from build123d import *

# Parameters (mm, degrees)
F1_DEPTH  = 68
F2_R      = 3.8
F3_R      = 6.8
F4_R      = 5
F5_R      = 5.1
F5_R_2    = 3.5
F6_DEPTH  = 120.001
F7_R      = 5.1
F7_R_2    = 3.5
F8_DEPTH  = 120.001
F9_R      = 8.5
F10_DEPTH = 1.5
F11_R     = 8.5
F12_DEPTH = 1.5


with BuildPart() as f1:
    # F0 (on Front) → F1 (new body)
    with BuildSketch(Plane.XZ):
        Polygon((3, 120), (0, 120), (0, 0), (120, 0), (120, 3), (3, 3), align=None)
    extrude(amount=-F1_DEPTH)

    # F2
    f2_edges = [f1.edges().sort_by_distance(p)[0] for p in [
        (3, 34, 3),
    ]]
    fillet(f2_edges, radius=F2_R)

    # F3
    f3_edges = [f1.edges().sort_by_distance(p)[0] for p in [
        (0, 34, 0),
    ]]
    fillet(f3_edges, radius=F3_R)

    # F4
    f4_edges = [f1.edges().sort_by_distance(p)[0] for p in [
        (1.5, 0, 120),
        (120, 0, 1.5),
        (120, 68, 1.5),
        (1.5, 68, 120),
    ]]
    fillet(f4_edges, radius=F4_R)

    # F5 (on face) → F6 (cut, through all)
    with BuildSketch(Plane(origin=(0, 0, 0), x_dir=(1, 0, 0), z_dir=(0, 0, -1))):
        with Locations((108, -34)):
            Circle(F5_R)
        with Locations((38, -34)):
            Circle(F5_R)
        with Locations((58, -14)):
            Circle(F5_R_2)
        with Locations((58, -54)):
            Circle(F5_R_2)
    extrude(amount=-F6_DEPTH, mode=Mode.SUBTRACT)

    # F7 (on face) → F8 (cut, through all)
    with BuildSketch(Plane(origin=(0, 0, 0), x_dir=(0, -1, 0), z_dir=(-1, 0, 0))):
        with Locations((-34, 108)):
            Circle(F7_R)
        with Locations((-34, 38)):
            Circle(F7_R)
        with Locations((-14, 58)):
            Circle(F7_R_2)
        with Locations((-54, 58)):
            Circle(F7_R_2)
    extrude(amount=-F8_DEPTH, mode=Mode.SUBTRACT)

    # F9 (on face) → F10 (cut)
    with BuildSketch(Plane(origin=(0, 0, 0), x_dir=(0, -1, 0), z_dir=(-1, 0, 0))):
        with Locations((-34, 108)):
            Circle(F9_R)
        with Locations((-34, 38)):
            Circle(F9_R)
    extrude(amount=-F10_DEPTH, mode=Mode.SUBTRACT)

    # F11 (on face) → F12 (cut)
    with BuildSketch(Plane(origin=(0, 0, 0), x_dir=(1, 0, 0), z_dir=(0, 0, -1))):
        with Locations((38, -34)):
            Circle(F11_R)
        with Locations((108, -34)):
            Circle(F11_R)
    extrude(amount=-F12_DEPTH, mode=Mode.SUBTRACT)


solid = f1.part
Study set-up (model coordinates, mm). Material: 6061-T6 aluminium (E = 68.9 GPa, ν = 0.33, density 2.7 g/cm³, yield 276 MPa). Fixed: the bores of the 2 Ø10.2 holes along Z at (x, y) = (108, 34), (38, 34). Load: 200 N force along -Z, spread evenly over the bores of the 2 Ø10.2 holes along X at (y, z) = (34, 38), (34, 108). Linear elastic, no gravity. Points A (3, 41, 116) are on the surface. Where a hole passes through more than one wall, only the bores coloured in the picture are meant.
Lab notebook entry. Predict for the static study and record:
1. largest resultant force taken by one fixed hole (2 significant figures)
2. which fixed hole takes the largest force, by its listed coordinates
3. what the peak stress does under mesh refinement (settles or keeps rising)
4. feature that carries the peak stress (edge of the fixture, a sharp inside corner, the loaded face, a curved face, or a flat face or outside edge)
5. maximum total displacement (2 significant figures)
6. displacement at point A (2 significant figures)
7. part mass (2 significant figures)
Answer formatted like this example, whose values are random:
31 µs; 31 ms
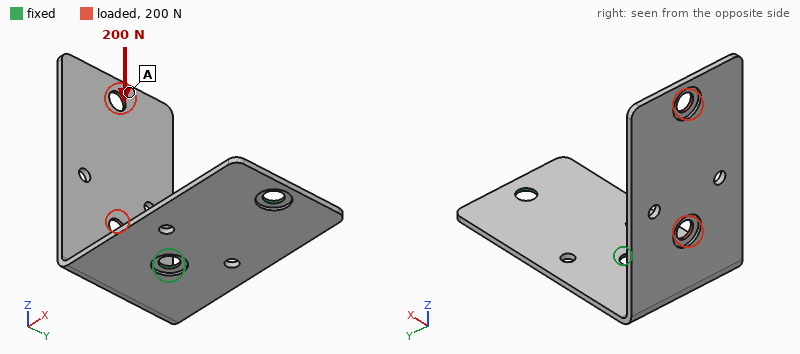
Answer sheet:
490 N; (38, 34); keeps rising; edge of the fixture; 1.9 mm; 1.8 mm; 120 g
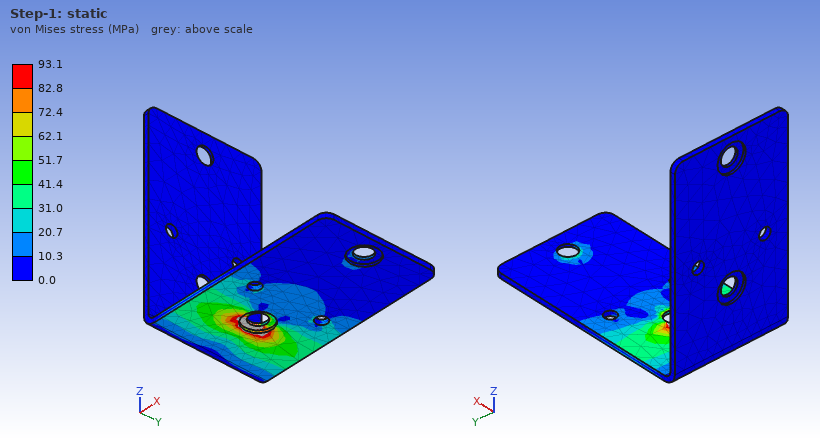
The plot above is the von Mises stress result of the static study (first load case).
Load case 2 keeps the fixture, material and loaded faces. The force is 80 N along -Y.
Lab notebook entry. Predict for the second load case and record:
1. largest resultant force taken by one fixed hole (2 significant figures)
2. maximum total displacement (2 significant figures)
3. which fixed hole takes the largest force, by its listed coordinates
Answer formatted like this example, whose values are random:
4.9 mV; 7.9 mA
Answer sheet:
140 N; 1.8 mm; (38, 34)
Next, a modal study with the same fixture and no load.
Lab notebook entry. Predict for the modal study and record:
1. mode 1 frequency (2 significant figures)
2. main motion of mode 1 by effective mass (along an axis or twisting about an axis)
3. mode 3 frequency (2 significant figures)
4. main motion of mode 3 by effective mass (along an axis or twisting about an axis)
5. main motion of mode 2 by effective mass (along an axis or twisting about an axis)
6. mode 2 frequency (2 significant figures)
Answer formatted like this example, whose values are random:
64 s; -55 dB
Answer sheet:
120 Hz; along X; 520 Hz; along Z; along Y; 180 Hz
